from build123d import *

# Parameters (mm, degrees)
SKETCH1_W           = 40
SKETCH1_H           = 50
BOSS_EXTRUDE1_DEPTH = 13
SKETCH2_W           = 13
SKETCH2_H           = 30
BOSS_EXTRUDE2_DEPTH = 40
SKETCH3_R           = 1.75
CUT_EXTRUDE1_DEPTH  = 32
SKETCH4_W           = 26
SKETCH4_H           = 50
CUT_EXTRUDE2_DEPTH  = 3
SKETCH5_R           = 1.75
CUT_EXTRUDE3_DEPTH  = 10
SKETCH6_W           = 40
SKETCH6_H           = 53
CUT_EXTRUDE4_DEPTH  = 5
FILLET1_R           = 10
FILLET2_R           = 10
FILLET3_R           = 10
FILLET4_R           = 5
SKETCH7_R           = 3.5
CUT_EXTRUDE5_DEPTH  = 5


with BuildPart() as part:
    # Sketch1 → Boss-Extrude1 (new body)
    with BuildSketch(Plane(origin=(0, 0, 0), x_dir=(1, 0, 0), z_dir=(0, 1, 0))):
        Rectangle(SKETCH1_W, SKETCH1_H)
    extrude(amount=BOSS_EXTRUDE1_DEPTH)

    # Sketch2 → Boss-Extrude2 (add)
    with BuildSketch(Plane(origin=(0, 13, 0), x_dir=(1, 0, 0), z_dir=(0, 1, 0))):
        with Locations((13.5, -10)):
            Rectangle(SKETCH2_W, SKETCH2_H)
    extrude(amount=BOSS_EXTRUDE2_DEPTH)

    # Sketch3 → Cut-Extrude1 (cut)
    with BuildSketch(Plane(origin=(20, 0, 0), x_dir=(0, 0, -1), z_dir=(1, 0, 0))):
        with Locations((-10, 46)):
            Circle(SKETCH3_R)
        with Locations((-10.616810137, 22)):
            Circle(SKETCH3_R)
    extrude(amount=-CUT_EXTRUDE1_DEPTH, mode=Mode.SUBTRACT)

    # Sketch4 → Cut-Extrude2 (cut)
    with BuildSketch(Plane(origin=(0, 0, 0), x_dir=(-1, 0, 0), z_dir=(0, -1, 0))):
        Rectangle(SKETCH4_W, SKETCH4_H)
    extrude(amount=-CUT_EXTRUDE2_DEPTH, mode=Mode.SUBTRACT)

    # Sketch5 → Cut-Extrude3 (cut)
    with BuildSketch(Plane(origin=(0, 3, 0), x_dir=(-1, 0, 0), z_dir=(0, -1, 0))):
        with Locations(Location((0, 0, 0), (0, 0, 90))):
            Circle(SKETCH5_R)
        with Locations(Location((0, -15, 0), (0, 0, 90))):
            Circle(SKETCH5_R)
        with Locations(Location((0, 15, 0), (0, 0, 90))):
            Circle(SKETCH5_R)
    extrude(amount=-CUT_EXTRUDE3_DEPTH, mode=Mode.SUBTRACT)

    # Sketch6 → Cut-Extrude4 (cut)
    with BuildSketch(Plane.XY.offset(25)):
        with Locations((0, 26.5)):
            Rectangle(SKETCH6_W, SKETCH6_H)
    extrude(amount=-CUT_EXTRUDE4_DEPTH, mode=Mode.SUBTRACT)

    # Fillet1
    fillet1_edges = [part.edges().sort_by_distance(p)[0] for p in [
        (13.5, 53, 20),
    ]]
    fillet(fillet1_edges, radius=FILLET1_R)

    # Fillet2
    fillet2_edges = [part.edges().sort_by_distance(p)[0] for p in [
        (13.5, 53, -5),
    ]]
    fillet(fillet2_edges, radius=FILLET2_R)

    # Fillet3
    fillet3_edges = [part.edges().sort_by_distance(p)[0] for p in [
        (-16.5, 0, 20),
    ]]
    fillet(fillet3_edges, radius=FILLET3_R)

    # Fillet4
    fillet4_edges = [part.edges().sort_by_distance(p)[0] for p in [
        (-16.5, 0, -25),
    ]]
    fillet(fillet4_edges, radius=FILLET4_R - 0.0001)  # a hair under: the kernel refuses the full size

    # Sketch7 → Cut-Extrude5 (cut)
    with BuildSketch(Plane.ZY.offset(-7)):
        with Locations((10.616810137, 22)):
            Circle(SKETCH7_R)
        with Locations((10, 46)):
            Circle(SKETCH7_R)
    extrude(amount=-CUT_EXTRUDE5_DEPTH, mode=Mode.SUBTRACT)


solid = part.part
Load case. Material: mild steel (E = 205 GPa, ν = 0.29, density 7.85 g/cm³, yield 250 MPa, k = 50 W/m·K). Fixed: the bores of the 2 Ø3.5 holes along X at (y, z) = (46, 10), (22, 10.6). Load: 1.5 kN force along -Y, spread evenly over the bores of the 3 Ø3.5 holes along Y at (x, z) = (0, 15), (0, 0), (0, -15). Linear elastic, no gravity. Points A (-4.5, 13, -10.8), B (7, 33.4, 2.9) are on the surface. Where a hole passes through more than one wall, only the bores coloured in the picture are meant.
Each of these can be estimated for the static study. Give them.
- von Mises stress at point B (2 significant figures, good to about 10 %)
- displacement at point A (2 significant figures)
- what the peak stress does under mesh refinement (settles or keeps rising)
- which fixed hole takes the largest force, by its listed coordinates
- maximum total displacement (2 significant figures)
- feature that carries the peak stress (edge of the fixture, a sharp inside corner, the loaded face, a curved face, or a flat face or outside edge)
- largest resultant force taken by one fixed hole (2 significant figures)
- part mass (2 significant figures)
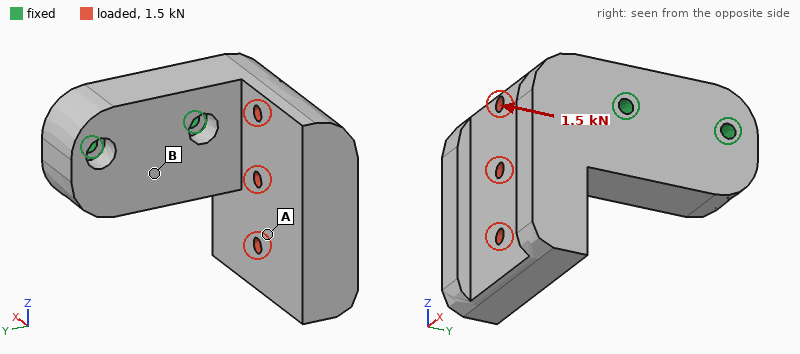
16 MPa
15 µm
keeps rising
(46, 10)
28 µm
edge of the fixture
1.4 kN
240 g
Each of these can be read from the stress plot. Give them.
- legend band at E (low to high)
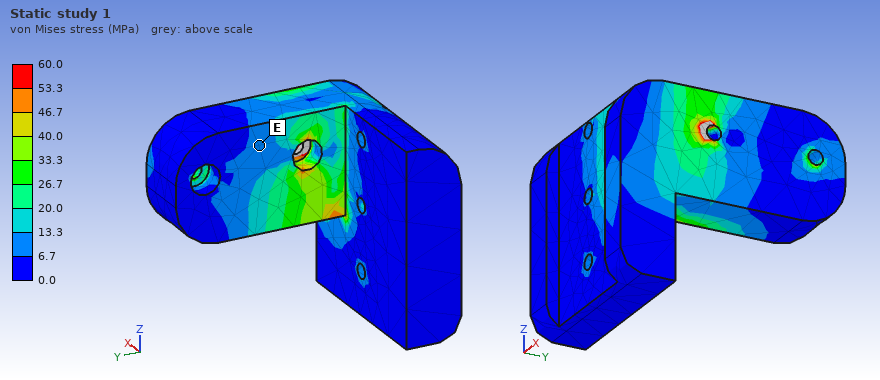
6.7 to 13.3 MPa
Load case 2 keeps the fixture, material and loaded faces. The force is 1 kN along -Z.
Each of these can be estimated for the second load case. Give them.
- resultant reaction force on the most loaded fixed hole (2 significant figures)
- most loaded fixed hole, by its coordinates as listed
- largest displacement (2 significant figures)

1.5 kN
(22, 10.6)
23 µm
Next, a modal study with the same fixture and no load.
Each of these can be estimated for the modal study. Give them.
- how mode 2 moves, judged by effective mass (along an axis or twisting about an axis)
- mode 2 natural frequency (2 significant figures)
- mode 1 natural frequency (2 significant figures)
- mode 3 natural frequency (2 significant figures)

along Y
3500 Hz
2700 Hz
6700 Hz
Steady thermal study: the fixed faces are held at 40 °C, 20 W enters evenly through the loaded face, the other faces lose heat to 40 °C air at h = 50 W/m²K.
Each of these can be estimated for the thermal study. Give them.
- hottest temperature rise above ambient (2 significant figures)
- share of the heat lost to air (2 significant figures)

28 K
33 %
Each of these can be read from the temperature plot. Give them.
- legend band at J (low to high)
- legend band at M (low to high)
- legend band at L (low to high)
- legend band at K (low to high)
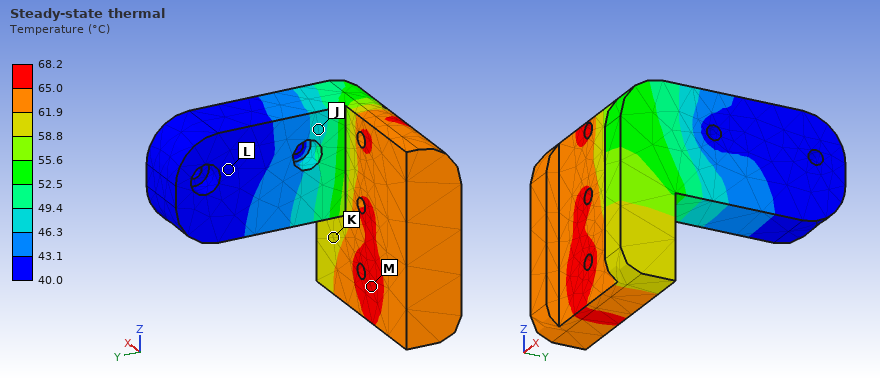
46.3 to 49.4 °C
65.0 to 68.2 °C
40.0 to 43.1 °C
58.8 to 61.9 °C
